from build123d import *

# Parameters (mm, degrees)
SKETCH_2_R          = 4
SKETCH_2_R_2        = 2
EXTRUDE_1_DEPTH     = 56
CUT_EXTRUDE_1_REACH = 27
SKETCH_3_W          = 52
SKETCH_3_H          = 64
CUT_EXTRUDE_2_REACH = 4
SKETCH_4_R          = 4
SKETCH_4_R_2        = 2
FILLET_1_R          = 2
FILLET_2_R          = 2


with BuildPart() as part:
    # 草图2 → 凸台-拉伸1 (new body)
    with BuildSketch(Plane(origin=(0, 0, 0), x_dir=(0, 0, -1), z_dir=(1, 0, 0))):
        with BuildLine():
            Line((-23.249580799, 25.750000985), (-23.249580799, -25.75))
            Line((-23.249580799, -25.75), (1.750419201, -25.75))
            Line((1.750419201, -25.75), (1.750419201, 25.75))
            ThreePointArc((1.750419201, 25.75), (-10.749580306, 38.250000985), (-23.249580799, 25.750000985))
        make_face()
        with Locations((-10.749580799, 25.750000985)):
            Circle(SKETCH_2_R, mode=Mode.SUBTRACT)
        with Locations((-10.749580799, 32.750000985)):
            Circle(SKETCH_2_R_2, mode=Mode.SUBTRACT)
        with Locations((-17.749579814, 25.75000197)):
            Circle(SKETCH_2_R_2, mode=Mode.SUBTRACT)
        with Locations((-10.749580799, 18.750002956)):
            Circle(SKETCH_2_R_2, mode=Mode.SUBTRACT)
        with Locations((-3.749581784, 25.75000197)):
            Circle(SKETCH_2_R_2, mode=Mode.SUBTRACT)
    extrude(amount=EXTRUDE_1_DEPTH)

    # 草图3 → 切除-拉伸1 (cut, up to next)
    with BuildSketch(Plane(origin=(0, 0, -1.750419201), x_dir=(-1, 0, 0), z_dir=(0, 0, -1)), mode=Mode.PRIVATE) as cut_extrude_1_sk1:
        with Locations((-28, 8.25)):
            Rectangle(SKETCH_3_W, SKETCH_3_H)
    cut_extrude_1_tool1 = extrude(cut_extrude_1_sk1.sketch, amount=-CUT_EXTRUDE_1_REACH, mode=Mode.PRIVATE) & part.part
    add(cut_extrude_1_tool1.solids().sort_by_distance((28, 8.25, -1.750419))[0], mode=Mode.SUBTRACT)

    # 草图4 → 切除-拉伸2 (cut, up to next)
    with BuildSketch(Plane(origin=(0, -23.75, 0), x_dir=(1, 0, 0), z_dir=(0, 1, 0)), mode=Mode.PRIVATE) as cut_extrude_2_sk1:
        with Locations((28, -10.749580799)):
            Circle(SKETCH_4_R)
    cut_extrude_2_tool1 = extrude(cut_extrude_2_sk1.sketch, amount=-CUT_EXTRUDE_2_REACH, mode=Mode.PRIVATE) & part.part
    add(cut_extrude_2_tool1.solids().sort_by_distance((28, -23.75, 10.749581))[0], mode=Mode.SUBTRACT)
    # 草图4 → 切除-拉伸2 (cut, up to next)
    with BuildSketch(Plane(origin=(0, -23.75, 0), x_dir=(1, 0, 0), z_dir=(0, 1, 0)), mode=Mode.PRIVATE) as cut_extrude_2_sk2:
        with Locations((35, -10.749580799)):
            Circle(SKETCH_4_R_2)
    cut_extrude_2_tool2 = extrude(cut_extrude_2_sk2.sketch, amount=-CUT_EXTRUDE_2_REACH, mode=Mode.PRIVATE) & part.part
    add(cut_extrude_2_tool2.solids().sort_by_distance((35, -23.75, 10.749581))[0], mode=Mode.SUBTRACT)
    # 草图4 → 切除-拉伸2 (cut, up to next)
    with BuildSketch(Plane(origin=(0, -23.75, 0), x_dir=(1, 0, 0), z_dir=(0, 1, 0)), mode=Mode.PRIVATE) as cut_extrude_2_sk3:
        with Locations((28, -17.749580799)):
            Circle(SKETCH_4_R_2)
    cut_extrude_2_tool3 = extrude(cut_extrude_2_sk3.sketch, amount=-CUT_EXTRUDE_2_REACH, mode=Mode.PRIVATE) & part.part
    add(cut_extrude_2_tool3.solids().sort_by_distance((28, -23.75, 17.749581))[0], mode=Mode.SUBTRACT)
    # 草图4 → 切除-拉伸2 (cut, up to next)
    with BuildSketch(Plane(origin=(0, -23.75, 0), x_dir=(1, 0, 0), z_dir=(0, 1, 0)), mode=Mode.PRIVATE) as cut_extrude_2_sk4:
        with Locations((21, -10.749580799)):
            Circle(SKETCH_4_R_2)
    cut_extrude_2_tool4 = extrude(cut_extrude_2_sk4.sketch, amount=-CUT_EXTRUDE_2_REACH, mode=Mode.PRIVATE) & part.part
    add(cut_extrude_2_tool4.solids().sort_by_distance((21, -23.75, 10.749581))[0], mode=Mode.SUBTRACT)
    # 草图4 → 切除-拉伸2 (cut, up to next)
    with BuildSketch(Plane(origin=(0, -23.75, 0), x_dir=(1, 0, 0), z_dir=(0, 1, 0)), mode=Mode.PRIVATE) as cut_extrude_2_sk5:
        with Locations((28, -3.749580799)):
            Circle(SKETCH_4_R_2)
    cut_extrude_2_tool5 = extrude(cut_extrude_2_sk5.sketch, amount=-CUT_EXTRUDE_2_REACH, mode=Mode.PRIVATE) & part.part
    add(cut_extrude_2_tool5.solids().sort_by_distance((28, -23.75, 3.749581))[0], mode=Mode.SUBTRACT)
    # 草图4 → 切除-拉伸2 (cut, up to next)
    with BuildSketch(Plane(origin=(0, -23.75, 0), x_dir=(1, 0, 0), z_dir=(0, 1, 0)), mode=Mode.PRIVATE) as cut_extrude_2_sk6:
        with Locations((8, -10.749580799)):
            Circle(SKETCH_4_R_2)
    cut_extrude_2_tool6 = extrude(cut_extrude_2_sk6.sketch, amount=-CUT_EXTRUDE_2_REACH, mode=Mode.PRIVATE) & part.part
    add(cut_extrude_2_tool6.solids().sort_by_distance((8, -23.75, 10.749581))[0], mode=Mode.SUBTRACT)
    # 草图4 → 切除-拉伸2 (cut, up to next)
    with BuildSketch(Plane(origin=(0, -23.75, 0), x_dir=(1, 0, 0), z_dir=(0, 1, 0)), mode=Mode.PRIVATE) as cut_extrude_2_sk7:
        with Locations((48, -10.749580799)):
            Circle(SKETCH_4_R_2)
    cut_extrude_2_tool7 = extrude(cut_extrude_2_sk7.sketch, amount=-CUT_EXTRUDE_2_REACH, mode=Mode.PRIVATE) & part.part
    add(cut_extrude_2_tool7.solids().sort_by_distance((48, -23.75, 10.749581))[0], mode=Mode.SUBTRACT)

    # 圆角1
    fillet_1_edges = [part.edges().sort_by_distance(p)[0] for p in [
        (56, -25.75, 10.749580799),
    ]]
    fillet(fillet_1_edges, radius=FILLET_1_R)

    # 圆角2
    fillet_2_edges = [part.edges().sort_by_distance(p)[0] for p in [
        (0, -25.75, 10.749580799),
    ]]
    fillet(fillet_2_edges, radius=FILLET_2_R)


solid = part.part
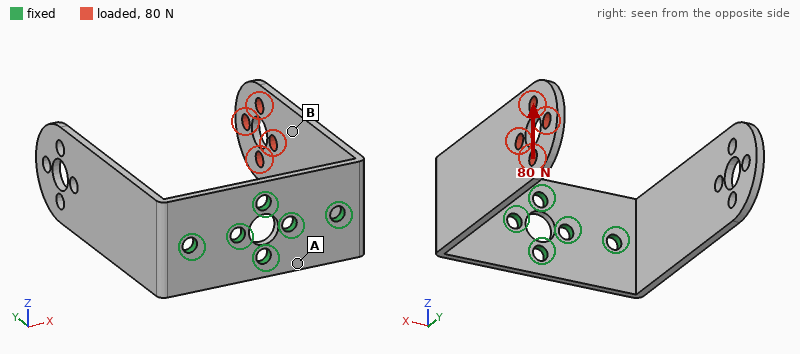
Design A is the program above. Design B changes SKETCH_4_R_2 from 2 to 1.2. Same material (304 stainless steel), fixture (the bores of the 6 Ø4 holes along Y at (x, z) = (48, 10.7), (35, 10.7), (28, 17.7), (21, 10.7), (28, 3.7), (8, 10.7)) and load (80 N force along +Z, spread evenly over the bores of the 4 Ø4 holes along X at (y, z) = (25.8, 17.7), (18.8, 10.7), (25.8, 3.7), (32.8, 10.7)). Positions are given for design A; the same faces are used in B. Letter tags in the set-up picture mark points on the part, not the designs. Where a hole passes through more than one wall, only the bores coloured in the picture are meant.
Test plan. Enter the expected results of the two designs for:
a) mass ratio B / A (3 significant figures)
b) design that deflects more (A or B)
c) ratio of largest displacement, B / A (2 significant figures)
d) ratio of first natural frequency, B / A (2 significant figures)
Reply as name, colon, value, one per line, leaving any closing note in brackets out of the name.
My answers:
mass ratio B / A: 1.01
design that deflects more: B
ratio of largest displacement, B / A: 1.3
ratio of first natural frequency, B / A: 0.97
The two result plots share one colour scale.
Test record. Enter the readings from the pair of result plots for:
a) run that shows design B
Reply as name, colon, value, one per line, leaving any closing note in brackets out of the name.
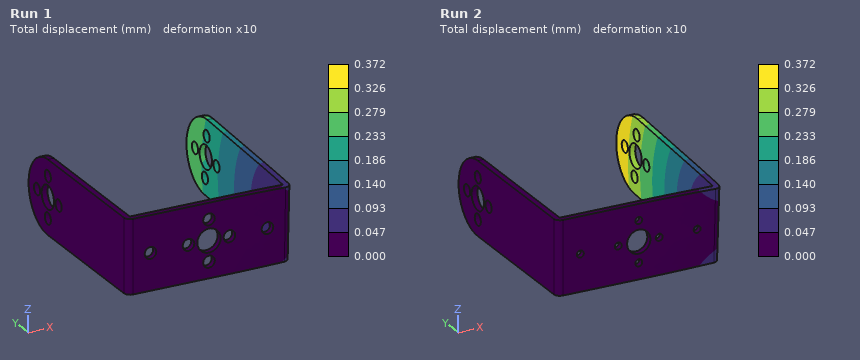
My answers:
run that shows design B: Run 2
